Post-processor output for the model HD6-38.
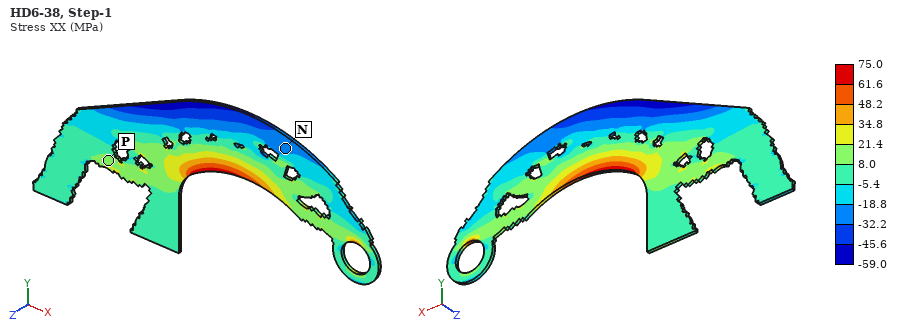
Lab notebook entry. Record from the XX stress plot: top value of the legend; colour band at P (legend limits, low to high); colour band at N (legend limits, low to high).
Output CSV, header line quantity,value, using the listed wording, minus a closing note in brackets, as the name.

quantity,value
top value of the legend,75.0 MPa
colour band at P,8.0 to 21.4 MPa
colour band at N,-32.2 to -18.8 MPa
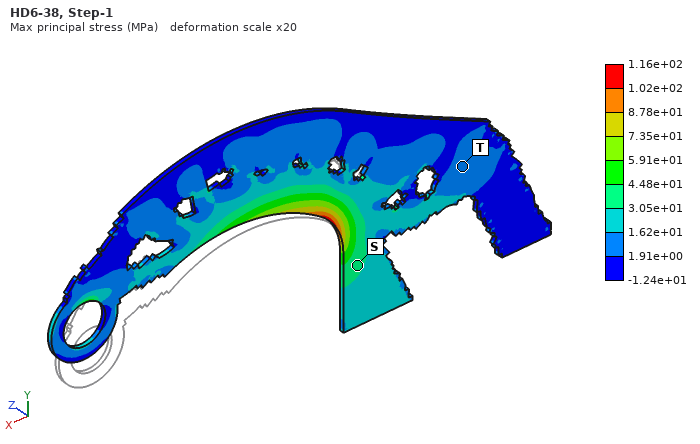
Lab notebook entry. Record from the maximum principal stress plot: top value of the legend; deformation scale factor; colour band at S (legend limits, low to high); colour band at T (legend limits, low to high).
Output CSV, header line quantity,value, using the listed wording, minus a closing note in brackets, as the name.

quantity,value
top value of the legend,1.16e+02 MPa
deformation scale factor,20
colour band at S,3.05e+01 to 4.48e+01 MPa
colour band at T,1.91e+00 to 1.62e+01 MPa
